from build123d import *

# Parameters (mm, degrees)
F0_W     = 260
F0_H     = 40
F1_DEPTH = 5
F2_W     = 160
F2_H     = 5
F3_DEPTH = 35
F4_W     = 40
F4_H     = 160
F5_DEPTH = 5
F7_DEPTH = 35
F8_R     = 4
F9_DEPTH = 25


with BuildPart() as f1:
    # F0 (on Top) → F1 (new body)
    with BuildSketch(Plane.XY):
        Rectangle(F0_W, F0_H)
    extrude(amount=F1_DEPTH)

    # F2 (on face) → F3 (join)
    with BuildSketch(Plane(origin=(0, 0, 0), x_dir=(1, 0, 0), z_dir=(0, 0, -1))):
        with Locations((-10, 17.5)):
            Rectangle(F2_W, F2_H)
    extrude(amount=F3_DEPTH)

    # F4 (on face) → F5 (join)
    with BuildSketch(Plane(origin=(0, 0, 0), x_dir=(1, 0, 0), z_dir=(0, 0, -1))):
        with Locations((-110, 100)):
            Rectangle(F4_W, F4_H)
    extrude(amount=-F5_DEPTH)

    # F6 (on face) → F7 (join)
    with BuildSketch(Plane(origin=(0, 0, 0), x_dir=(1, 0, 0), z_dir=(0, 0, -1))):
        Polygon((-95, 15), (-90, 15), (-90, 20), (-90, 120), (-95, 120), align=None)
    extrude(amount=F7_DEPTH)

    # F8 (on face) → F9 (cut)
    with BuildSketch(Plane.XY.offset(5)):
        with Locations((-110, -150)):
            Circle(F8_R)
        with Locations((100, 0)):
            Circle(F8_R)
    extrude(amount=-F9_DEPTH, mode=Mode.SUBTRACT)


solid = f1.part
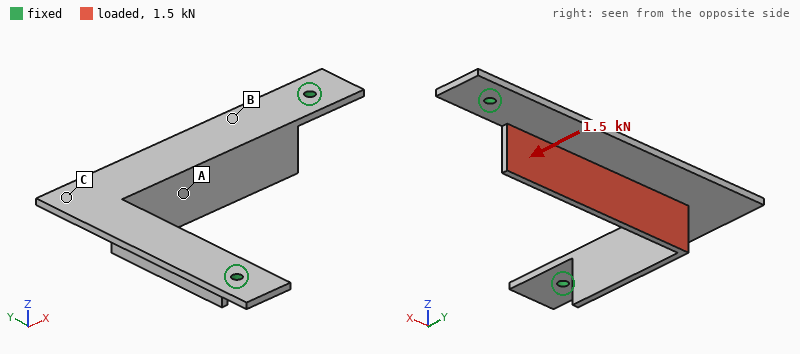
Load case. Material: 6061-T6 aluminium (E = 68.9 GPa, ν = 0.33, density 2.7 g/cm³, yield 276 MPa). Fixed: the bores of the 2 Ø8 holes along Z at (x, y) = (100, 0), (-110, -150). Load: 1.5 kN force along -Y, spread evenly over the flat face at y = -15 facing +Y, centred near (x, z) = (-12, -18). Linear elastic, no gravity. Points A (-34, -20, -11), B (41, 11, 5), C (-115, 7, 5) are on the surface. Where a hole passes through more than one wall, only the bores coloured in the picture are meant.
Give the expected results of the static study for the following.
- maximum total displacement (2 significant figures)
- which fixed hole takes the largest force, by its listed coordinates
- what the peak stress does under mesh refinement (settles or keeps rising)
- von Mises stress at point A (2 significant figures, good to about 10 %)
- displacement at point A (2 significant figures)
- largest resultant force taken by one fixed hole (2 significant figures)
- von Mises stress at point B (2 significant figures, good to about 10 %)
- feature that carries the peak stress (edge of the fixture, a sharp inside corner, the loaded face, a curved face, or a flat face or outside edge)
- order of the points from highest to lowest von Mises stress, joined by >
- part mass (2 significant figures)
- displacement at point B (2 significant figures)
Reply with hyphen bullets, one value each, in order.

- 1.8 mm
- (-110, -150)
- keeps rising
- 19 MPa
- 0.72 mm
- 910 N
- 36 MPa
- edge of the fixture
- B > A > C
- 350 g
- 0.53 mm
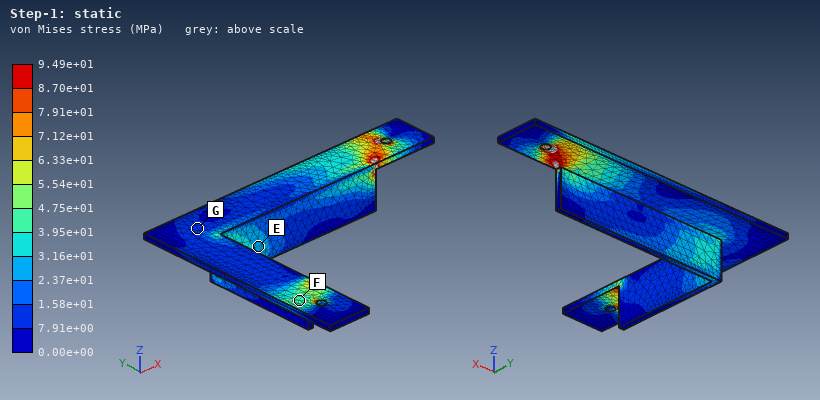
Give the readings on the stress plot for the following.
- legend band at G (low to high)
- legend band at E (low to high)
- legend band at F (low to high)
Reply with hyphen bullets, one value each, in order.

- 7.91e+00 to 1.58e+01 MPa
- 2.37e+01 to 3.16e+01 MPa
- 3.95e+01 to 4.75e+01 MPa
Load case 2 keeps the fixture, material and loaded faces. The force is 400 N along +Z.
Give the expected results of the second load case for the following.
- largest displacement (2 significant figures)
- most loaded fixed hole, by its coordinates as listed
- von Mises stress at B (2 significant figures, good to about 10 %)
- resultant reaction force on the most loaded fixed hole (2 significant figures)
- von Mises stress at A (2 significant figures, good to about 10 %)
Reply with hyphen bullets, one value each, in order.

- 2.2 mm
- (100, 0)
- 20 MPa
- 270 N
- 17 MPa
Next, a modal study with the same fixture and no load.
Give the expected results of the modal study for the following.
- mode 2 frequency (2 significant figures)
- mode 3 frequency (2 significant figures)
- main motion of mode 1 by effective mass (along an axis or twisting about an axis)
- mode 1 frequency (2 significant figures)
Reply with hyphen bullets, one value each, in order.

- 1000 Hz
- 1200 Hz
- along Z
- 160 Hz
